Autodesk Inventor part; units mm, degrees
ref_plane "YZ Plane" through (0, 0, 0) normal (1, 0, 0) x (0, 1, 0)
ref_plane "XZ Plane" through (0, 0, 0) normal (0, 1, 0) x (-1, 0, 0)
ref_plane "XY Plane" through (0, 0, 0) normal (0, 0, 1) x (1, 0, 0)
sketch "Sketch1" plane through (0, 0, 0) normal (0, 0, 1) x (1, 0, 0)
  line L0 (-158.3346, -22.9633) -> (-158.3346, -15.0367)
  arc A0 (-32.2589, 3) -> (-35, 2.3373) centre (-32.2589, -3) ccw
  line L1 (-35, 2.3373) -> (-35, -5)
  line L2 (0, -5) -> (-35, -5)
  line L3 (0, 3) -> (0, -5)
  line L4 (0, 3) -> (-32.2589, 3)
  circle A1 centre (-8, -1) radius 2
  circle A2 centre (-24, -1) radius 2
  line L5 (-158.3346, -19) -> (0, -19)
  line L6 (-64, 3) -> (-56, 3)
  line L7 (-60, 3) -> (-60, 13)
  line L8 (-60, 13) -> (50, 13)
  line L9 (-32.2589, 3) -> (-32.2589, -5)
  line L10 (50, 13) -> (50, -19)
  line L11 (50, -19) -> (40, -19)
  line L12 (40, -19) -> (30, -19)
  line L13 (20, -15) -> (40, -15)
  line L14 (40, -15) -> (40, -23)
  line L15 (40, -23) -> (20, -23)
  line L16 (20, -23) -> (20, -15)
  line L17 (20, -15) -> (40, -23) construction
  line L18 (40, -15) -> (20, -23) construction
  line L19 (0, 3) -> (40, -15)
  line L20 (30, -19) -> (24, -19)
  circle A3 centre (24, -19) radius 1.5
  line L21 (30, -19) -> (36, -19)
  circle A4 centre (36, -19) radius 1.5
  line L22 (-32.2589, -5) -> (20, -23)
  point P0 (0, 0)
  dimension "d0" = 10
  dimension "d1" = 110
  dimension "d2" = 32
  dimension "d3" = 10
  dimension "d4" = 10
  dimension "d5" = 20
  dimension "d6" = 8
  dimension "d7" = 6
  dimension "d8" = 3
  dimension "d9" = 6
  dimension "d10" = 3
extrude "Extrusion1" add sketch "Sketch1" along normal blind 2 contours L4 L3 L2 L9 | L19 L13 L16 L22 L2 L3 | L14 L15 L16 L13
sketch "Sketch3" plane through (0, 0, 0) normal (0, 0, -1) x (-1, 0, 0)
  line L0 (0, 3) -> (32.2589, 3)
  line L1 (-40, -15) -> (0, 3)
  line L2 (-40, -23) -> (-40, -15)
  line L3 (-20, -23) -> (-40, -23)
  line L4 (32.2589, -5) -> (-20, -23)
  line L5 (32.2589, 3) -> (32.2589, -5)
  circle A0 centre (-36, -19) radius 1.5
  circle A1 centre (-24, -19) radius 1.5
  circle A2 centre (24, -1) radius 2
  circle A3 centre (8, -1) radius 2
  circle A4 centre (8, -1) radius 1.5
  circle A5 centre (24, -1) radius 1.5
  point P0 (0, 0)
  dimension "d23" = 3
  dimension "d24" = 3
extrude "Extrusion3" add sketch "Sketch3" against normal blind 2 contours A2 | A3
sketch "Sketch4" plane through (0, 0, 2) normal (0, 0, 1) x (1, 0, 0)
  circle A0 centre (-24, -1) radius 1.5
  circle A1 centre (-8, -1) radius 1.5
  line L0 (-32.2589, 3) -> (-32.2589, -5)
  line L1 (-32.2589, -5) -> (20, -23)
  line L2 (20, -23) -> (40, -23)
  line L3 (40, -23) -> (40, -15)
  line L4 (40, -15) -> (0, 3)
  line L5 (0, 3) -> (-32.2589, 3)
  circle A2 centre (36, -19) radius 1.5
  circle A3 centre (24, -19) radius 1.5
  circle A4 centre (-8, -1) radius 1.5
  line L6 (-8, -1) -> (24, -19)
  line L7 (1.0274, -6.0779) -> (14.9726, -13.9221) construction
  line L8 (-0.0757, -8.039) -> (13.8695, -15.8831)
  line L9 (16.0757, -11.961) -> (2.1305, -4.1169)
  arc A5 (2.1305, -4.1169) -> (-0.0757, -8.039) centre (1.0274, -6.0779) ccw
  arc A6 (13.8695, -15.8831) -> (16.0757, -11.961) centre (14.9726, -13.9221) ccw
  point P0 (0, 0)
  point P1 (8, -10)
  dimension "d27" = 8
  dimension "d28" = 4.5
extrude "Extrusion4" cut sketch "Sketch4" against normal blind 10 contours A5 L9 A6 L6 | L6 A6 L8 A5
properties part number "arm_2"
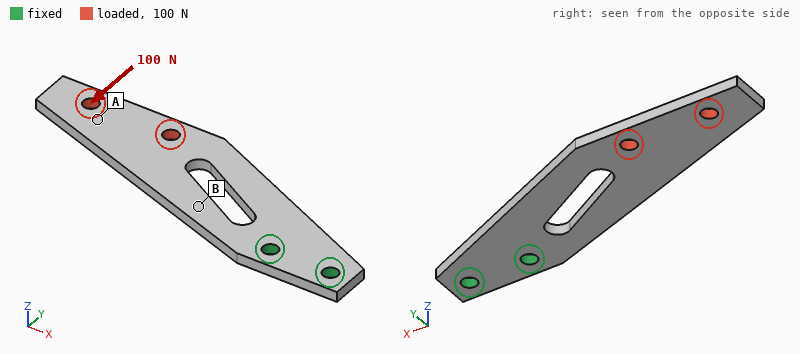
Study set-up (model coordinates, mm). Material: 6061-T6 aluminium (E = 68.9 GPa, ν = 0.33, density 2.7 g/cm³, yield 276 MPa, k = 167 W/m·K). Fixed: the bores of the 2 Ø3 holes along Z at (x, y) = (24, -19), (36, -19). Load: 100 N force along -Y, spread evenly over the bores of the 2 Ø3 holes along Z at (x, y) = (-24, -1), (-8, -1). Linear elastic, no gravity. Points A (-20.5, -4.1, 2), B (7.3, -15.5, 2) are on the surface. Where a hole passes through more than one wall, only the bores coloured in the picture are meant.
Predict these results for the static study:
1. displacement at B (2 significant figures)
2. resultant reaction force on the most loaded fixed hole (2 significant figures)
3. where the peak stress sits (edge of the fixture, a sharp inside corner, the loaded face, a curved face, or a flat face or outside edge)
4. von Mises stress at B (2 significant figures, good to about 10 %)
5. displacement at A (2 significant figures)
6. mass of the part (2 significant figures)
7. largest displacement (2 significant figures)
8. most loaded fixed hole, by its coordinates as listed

0.037 mm
380 N
edge of the fixture
21 MPa
0.12 mm
5.0 g
0.16 mm
(24, -19)
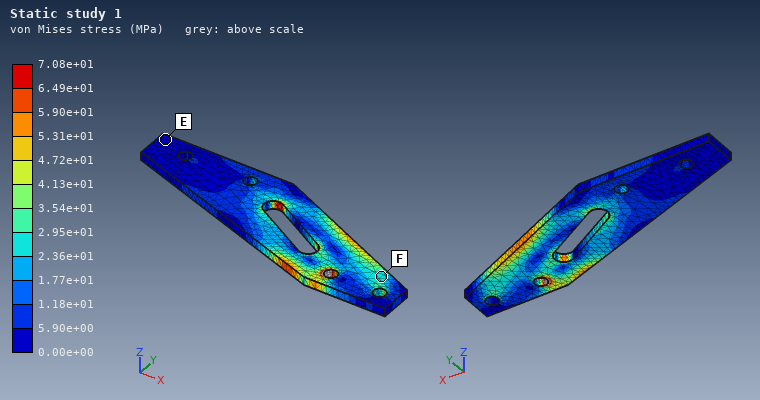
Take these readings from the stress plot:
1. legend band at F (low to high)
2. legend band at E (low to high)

2.36e+01 to 2.95e+01 MPa
0.00e+00 to 5.90e+00 MPa
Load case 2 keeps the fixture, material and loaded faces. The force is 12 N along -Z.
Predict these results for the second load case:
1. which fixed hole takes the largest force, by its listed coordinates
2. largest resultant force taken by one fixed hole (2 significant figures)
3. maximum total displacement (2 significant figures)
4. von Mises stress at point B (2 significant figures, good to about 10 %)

(24, -19)
27 N
0.85 mm
40 MPa
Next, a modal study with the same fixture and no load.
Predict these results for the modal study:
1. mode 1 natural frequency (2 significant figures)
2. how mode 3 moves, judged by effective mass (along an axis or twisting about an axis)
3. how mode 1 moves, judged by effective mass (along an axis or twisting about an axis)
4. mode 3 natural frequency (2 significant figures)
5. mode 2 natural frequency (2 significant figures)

510 Hz
along Y
along Z
3000 Hz
2800 Hz
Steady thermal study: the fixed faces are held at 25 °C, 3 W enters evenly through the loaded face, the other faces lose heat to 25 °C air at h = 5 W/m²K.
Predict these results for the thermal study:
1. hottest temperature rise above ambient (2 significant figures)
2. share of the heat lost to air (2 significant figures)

30 K
5.6 %
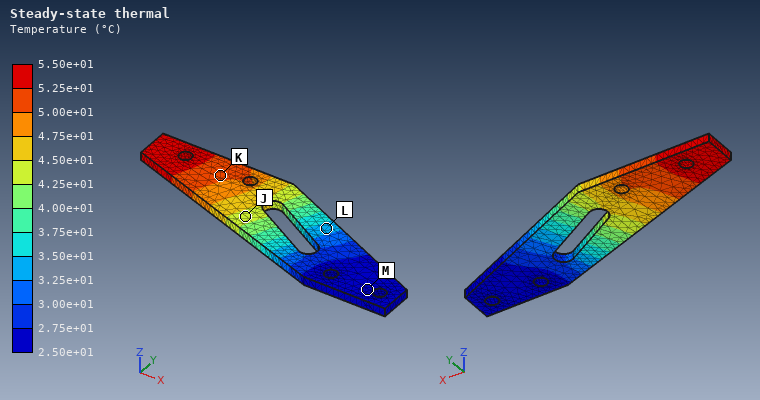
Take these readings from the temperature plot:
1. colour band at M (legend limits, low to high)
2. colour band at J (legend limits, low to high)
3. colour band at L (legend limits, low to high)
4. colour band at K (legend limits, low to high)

2.50e+01 to 2.75e+01 °C
4.25e+01 to 4.50e+01 °C
3.25e+01 to 3.50e+01 °C
5.00e+01 to 5.25e+01 °C
